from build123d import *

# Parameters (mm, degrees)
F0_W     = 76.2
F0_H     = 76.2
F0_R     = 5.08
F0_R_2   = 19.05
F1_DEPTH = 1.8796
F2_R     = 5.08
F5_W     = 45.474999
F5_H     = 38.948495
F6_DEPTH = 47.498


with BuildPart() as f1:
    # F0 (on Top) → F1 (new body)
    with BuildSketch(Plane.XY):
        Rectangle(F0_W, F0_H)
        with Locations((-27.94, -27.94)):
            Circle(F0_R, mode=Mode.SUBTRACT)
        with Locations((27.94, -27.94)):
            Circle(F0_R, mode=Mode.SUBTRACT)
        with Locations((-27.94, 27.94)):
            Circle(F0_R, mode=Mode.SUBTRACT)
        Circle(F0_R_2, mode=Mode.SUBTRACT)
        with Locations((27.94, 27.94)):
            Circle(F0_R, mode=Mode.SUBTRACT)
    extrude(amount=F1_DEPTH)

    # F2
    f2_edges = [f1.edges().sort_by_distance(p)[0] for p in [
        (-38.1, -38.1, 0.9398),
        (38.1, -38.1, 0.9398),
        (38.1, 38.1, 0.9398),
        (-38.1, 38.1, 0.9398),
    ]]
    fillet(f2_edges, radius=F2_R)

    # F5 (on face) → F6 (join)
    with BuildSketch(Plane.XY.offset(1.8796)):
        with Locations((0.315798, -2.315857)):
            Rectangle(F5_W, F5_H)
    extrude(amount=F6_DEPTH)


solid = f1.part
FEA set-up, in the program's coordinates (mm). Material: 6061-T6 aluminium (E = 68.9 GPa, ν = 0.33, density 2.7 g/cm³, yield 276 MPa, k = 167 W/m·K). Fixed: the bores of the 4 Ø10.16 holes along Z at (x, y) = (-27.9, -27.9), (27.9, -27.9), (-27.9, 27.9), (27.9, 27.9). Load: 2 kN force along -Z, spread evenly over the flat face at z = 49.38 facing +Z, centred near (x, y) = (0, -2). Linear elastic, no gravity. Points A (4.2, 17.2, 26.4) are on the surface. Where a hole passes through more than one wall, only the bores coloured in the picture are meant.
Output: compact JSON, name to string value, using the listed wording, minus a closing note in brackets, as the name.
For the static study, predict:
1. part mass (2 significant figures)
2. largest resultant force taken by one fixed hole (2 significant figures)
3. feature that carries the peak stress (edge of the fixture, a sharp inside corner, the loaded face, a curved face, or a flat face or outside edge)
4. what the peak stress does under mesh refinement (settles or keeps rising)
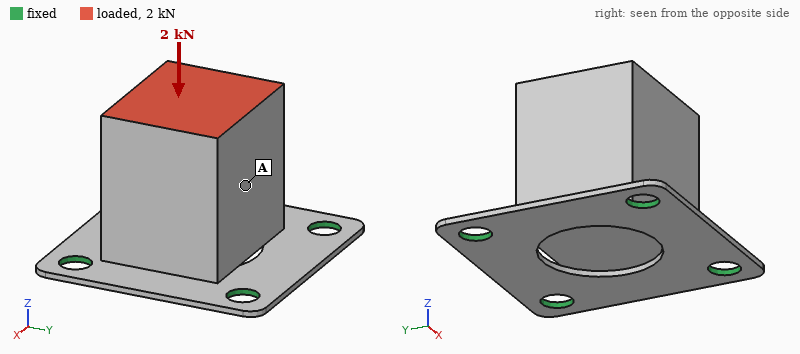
{"part mass": "250 g", "largest resultant force taken by one fixed hole": "640 N", "feature that carries the peak stress": "edge of the fixture", "what the peak stress does under mesh refinement": "keeps rising"}
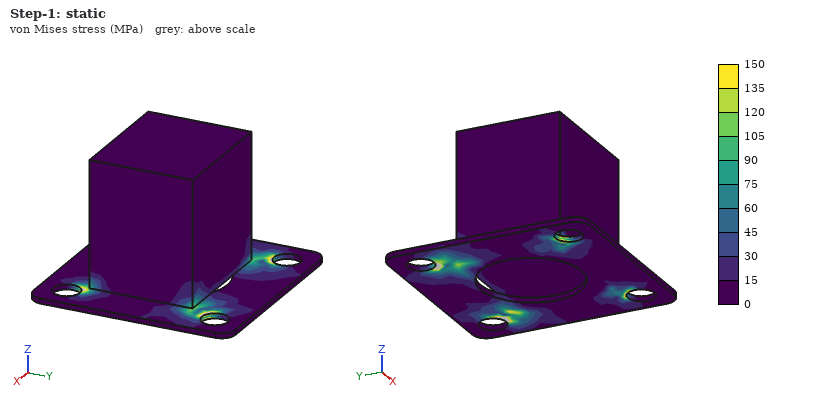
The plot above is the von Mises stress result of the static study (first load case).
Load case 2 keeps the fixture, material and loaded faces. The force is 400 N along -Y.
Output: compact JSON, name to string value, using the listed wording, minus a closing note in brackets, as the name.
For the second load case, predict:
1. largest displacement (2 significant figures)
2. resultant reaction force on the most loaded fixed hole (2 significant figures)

{"largest displacement": "50 µm", "resultant reaction force on the most loaded fixed hole": "270 N"}
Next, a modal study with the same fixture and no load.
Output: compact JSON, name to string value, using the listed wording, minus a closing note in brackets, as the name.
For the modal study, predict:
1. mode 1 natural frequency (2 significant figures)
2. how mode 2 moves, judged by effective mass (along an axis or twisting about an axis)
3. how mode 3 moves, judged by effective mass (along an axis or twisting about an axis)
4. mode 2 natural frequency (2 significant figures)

{"mode 1 natural frequency": "1500 Hz", "how mode 2 moves, judged by effective mass": "along X", "how mode 3 moves, judged by effective mass": "along Z", "mode 2 natural frequency": "1900 Hz"}
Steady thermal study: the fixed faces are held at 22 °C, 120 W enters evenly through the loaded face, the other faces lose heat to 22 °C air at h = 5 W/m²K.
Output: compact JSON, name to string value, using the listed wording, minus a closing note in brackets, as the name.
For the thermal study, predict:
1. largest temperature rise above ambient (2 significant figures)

{"largest temperature rise above ambient": "64 K"}
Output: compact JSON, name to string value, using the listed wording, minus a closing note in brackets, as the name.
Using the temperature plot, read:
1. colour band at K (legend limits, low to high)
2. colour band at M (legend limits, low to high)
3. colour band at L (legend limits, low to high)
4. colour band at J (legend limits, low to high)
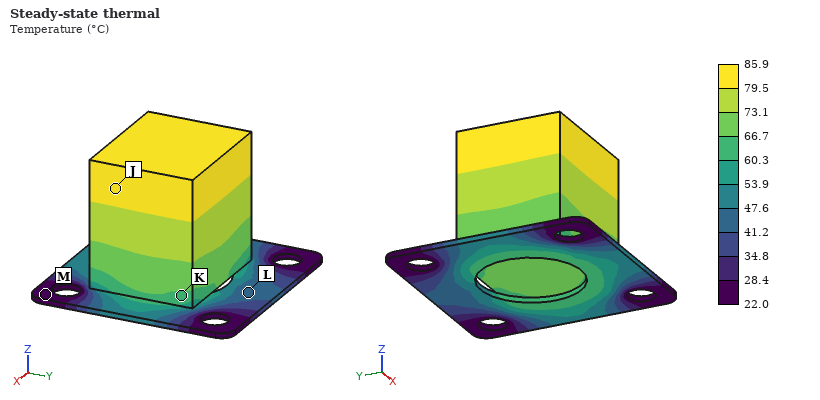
{"colour band at K": "60.3 to 66.7 °C", "colour band at M": "22.0 to 28.4 °C", "colour band at L": "41.2 to 47.6 °C", "colour band at J": "79.5 to 85.9 °C"}
